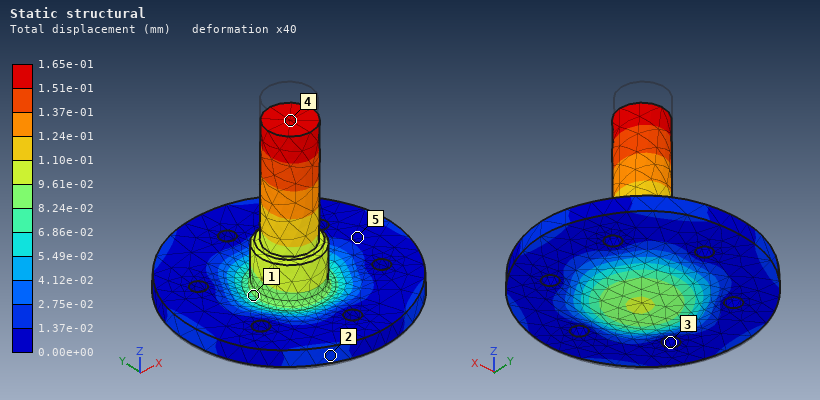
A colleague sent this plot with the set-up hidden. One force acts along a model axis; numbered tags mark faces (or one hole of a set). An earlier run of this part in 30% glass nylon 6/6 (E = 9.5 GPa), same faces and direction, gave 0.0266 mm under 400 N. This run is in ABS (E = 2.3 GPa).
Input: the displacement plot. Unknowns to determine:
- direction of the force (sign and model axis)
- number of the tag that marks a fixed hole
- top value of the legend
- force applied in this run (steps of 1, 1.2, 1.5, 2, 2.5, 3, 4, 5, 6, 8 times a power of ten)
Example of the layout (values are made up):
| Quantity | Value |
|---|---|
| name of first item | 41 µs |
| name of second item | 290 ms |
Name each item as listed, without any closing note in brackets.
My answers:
| Quantity | Value |
|---|---|
| direction of the force | -Z |
| number of the tag that marks a fixed hole | 3 |
| top value of the legend | 1.65e-01 mm |
| force applied in this run | 600 N |
